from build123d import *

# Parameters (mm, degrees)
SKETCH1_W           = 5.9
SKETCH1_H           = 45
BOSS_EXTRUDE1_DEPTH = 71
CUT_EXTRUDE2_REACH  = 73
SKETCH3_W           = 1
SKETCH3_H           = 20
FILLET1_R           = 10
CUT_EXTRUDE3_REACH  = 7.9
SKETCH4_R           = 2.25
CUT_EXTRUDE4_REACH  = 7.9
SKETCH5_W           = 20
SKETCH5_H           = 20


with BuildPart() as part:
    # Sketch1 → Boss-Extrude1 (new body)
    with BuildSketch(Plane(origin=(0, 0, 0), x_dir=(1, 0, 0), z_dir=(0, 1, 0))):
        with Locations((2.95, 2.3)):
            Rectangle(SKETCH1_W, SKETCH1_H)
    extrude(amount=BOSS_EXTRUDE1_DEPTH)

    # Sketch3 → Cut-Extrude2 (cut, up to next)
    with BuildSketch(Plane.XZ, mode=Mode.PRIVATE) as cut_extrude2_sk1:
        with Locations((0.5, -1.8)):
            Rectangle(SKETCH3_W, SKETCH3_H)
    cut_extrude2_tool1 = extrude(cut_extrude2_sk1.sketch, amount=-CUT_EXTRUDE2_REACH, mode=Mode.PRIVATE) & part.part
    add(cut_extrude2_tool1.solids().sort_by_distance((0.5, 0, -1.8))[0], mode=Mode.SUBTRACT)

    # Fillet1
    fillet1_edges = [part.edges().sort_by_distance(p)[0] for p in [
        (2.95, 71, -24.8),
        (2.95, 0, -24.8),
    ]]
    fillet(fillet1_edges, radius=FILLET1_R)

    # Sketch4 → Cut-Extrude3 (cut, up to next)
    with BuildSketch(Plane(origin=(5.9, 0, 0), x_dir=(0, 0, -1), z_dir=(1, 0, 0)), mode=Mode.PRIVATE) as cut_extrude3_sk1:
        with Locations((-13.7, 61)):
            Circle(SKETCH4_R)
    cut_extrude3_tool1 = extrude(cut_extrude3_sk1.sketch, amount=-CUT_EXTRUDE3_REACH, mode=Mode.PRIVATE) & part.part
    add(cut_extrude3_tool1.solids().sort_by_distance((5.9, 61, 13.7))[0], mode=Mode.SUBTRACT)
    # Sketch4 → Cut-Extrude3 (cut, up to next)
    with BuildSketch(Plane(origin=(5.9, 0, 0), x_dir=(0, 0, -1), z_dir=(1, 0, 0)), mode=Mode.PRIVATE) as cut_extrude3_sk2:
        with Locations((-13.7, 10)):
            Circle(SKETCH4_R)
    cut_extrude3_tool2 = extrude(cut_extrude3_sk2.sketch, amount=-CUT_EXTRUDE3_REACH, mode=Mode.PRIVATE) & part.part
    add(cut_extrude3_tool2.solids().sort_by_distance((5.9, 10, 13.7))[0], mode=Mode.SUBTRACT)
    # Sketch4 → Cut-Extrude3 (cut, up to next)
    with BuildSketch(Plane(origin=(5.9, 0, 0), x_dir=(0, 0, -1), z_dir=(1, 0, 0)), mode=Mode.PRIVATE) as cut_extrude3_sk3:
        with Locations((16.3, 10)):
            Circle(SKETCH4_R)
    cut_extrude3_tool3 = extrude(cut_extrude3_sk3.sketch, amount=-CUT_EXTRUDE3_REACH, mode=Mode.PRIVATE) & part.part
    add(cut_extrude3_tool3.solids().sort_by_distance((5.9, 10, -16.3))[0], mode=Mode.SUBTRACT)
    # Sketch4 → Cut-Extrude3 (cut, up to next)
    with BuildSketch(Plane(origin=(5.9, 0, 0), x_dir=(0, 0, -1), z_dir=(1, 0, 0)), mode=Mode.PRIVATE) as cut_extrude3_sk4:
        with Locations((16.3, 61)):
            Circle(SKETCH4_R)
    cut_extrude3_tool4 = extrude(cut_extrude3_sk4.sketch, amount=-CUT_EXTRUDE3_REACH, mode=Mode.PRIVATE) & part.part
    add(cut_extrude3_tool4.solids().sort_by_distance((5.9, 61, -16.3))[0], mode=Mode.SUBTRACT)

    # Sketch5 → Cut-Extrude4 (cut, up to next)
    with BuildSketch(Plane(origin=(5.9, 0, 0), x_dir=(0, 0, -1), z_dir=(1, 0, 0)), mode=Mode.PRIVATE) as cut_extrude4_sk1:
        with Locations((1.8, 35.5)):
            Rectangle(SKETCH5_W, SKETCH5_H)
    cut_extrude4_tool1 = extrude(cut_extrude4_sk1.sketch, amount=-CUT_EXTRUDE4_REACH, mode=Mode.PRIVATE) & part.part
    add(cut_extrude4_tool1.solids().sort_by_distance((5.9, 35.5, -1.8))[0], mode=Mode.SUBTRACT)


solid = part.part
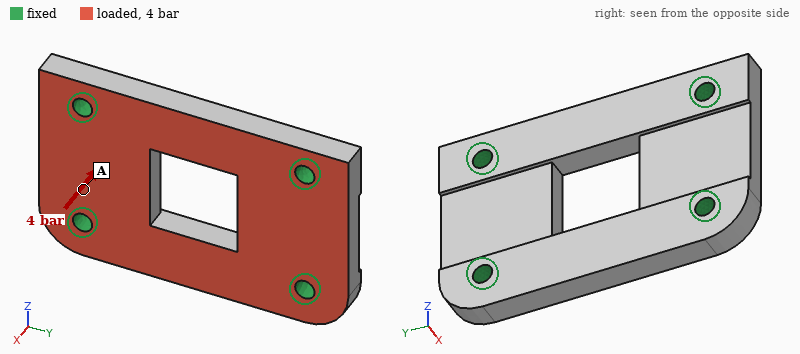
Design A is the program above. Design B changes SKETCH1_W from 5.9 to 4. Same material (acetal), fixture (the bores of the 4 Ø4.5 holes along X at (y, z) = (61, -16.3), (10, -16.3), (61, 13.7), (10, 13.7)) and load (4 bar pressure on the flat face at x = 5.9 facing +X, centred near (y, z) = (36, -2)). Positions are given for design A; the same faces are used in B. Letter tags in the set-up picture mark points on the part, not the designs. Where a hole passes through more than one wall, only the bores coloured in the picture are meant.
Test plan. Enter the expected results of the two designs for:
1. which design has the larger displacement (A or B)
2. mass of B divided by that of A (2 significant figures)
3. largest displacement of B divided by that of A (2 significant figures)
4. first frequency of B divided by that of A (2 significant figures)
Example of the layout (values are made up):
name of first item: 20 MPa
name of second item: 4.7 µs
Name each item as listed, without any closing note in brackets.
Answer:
which design has the larger displacement: B
mass of B divided by that of A: 0.72
largest displacement of B divided by that of A: 2.6
first frequency of B divided by that of A: 0.74
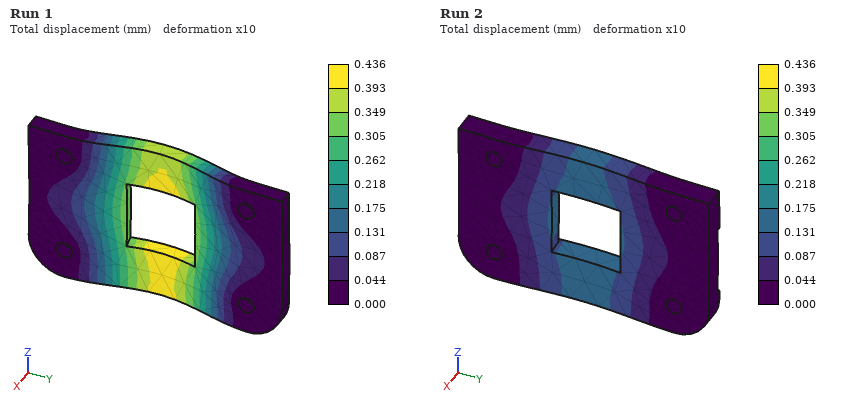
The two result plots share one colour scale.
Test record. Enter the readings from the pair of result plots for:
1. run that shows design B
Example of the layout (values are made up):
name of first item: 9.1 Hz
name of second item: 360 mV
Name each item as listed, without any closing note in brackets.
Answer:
run that shows design B: Run 1
